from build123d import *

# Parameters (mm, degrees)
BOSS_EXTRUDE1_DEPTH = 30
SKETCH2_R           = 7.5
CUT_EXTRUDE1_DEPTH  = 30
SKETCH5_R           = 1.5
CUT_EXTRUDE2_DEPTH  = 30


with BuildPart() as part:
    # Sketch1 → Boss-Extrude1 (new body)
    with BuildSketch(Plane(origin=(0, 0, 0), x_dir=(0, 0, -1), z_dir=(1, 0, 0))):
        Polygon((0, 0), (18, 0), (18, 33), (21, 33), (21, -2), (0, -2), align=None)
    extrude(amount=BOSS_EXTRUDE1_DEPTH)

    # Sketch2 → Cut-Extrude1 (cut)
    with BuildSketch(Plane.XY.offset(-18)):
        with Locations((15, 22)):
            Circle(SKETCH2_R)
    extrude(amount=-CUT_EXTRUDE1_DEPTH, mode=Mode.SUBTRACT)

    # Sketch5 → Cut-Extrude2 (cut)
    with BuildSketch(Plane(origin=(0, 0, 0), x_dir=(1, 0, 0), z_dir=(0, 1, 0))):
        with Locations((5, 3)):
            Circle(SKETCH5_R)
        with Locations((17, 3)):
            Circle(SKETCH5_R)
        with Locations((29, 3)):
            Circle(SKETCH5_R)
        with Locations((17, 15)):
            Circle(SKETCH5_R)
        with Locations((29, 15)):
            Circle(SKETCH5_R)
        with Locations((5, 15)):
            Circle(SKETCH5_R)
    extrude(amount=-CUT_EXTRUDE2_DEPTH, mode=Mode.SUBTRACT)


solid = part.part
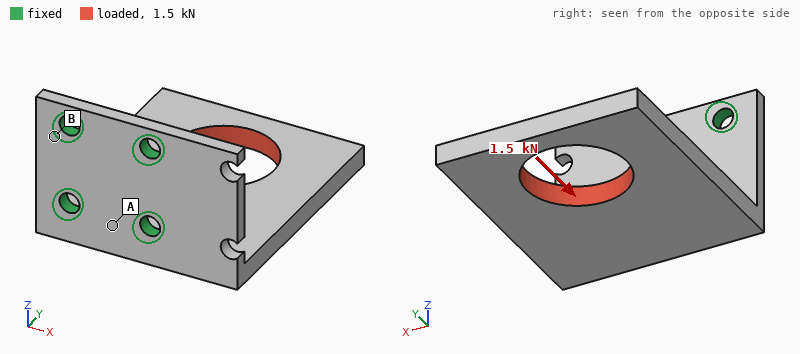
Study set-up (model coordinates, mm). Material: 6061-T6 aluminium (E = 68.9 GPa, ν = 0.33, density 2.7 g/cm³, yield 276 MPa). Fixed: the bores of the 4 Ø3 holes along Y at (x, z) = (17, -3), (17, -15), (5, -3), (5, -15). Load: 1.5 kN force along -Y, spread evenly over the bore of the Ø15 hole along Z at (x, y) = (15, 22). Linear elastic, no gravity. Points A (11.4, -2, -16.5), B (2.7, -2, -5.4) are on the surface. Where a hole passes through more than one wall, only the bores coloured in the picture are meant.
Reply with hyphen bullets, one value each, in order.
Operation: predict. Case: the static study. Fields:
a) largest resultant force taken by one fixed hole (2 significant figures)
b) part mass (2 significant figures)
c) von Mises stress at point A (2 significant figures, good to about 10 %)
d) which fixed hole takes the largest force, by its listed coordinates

- 1.2 kN
- 9.8 g
- 110 MPa
- (17, -15)
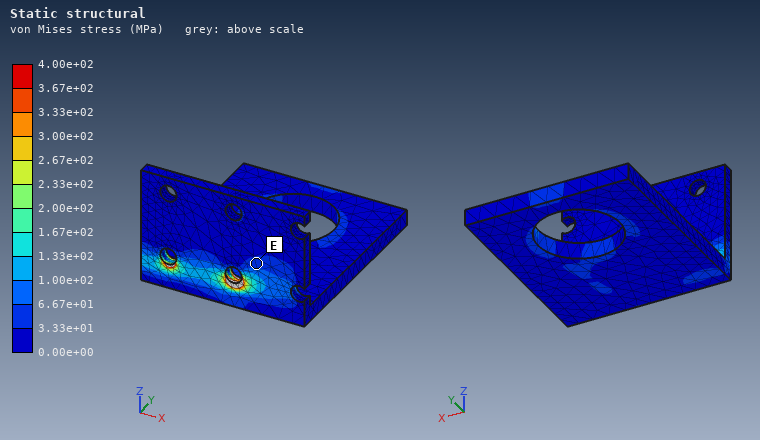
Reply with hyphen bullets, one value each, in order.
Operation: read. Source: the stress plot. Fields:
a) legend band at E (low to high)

- 3.33e+01 to 6.67e+01 MPa
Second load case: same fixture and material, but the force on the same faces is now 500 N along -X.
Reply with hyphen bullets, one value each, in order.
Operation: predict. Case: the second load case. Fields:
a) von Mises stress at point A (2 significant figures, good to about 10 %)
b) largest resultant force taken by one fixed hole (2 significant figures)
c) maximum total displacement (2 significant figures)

- 30 MPa
- 880 N
- 0.17 mm
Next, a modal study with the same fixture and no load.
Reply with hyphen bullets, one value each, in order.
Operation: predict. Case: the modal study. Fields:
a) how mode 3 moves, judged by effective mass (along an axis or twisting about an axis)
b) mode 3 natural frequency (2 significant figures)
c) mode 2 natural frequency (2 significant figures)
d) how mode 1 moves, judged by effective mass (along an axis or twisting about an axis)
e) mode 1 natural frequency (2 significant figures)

- along X
- 5500 Hz
- 4100 Hz
- along Z
- 1500 Hz
